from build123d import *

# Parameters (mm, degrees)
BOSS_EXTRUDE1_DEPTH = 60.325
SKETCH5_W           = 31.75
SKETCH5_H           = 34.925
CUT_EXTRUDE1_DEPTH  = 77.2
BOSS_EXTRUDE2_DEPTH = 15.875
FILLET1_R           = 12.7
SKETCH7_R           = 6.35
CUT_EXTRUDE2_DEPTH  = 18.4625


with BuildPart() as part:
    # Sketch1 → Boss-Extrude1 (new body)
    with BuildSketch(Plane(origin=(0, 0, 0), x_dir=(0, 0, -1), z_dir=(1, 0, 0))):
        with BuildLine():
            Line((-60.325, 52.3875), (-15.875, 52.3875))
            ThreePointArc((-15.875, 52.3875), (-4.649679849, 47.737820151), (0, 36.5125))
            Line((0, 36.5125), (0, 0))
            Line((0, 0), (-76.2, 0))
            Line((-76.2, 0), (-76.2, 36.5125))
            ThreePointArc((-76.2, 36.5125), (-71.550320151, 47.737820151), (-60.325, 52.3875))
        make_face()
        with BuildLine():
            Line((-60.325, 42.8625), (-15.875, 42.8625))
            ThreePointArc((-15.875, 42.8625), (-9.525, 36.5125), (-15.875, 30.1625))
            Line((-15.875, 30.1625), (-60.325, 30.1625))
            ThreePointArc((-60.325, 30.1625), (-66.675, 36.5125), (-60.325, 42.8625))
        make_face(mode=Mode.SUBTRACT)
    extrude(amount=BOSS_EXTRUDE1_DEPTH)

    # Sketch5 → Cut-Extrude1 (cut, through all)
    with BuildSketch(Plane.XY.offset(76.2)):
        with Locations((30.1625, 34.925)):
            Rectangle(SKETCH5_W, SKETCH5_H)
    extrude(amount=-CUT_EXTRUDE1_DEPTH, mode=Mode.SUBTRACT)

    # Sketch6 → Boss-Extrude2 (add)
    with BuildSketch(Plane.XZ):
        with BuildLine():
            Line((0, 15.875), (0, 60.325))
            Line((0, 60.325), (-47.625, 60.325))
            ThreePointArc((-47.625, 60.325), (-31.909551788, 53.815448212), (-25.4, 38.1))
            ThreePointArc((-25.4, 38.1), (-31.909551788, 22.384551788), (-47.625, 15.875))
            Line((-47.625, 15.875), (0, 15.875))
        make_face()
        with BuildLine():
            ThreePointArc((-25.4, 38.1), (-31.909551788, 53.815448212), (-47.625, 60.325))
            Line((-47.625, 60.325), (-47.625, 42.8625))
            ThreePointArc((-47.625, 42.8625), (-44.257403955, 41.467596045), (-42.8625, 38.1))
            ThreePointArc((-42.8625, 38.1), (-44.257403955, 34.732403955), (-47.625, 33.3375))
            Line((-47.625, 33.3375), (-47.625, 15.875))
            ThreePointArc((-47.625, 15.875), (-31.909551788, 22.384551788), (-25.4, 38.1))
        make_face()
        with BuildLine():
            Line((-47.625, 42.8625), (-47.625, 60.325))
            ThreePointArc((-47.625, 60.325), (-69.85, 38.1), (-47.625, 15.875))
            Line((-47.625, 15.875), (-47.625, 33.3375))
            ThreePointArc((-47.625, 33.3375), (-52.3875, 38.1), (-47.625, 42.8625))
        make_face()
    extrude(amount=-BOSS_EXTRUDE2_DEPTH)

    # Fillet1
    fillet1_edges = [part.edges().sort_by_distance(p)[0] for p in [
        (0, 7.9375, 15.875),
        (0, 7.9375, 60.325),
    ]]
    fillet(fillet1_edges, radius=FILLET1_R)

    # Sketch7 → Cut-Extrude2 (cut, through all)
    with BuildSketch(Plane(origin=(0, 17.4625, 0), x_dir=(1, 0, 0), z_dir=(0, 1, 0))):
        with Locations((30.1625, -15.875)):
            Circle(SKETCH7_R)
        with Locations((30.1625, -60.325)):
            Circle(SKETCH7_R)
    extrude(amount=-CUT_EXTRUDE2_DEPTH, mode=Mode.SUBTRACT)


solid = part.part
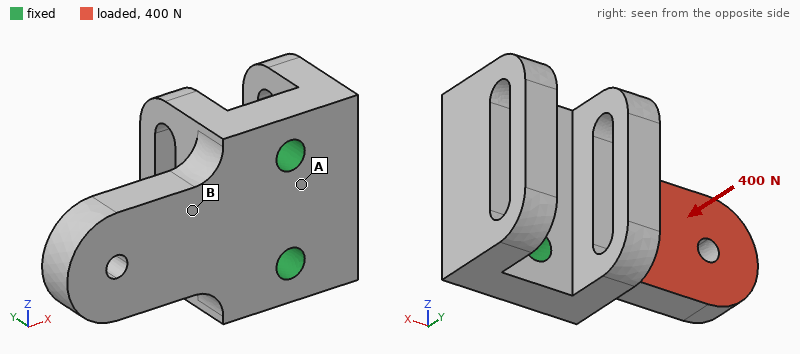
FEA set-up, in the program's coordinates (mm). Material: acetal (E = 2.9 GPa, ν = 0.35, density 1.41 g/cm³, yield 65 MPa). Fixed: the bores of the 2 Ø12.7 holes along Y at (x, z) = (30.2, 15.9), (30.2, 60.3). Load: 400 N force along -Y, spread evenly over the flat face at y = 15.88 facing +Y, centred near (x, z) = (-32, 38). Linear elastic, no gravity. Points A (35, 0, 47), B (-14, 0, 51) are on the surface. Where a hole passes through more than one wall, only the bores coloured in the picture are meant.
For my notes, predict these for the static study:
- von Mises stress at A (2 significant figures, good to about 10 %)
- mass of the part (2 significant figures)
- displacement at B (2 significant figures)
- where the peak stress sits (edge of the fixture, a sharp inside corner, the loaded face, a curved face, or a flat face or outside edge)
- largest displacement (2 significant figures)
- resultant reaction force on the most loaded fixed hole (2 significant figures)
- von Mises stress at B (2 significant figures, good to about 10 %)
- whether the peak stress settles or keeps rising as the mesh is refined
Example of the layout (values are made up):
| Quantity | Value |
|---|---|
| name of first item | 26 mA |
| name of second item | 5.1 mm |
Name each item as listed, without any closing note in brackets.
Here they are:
| Quantity | Value |
|---|---|
| von Mises stress at A | 1.5 MPa |
| mass of the part | 250 g |
| displacement at B | 0.21 mm |
| where the peak stress sits | edge of the fixture |
| largest displacement | 0.82 mm |
| resultant reaction force on the most loaded fixed hole | 200 N |
| von Mises stress at B | 4.0 MPa |
| whether the peak stress settles or keeps rising as the mesh is refined | keeps rising |
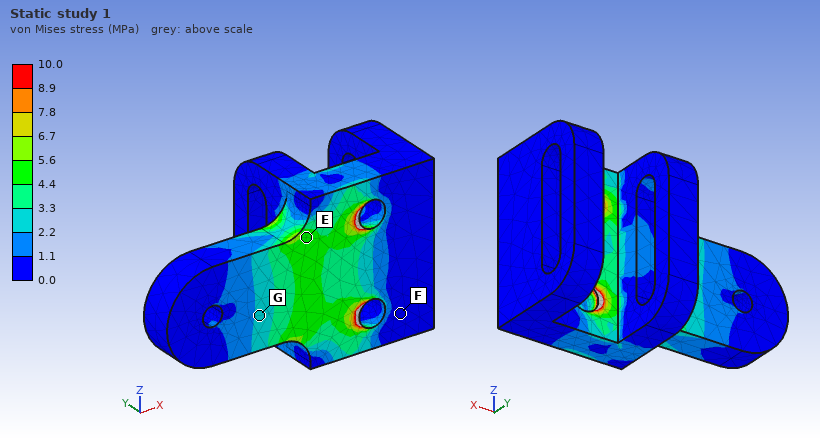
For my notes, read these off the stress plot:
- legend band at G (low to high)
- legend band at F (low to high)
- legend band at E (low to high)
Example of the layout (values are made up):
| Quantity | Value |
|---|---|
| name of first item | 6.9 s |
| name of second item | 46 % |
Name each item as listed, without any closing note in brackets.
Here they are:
| Quantity | Value |
|---|---|
| legend band at G | 2.2 to 3.3 MPa |
| legend band at F | 0.0 to 1.1 MPa |
| legend band at E | 4.4 to 5.6 MPa |
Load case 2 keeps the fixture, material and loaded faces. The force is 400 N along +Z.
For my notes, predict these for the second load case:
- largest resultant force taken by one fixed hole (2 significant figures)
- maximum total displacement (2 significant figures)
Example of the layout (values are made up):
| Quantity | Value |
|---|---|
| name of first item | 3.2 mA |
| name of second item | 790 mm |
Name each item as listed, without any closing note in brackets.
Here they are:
| Quantity | Value |
|---|---|
| largest resultant force taken by one fixed hole | 510 N |
| maximum total displacement | 0.12 mm |
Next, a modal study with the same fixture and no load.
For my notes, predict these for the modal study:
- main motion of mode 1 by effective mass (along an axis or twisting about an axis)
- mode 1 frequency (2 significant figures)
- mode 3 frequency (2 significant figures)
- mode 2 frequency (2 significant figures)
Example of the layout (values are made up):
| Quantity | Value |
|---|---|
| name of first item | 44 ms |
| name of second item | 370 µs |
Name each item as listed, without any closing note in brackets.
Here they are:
| Quantity | Value |
|---|---|
| main motion of mode 1 by effective mass | along Y |
| mode 1 frequency | 540 Hz |
| mode 3 frequency | 1300 Hz |
| mode 2 frequency | 1200 Hz |
